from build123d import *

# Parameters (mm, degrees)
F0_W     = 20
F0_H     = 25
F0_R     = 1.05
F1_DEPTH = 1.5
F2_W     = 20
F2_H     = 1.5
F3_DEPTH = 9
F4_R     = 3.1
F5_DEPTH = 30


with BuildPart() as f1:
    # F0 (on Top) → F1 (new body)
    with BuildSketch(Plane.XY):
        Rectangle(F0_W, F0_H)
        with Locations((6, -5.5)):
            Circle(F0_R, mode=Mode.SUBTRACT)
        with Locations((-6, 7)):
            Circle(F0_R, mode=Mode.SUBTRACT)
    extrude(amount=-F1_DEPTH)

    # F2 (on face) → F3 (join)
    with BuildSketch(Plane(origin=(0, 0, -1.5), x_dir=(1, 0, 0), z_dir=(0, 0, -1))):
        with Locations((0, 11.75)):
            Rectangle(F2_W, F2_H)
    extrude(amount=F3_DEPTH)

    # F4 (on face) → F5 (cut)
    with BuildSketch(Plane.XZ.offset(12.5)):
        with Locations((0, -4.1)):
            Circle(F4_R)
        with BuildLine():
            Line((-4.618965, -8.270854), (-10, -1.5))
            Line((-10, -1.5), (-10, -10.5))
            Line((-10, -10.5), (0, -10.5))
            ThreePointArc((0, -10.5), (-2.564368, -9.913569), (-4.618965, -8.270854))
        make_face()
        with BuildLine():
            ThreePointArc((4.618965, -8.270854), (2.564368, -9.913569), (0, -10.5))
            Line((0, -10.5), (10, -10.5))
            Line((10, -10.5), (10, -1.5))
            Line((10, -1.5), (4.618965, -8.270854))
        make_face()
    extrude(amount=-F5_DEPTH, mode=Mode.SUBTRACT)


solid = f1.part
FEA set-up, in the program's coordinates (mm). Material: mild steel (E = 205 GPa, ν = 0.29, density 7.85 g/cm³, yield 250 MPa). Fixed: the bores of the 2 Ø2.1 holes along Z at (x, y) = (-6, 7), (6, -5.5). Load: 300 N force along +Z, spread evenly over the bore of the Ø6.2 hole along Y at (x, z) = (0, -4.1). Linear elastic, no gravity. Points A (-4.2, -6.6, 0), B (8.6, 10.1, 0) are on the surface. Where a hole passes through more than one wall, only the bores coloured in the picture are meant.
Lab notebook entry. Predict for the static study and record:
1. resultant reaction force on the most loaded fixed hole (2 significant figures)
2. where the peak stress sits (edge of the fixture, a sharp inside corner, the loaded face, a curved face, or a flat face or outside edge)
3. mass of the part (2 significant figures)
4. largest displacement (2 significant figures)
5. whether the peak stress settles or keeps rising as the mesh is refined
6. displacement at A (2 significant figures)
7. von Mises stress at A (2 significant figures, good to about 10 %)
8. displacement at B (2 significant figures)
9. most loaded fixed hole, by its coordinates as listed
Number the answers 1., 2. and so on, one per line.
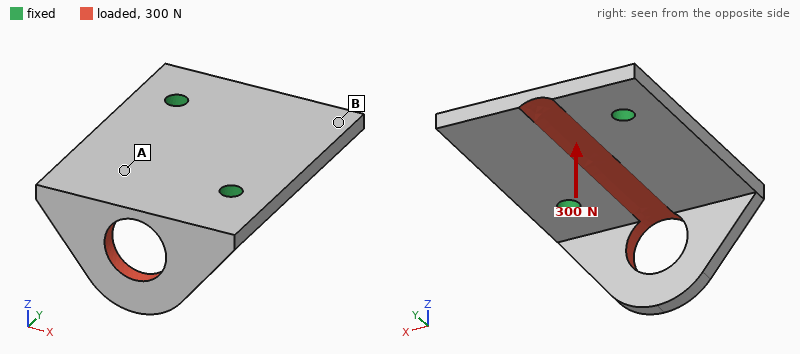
1. 190 N
2. edge of the fixture
3. 6.6 g
4. 54 µm
5. keeps rising
6. 22 µm
7. 44 MPa
8. 8.6 µm
9. (6, -5.5)
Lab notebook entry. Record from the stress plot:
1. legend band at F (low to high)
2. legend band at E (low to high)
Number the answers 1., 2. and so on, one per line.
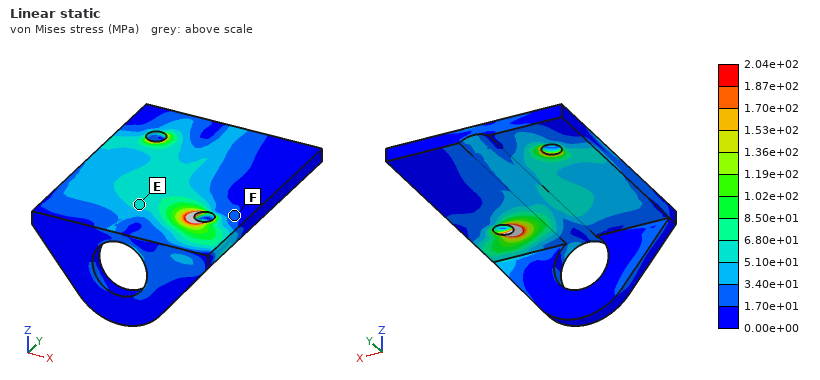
1. 1.70e+01 to 3.40e+01 MPa
2. 5.10e+01 to 6.80e+01 MPa
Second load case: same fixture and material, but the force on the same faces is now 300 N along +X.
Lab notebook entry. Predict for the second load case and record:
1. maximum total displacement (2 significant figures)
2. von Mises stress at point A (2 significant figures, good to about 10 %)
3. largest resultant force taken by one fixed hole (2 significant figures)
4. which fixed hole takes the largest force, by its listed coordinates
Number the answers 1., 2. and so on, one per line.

1. 19 µm
2. 13 MPa
3. 190 N
4. (6, -5.5)
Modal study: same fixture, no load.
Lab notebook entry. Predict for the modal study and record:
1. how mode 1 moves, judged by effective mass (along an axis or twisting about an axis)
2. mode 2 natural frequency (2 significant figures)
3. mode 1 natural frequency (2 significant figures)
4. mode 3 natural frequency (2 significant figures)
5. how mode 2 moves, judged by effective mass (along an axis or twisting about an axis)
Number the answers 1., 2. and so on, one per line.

1. along Z
2. 8100 Hz
3. 5500 Hz
4. 9900 Hz
5. along Z
